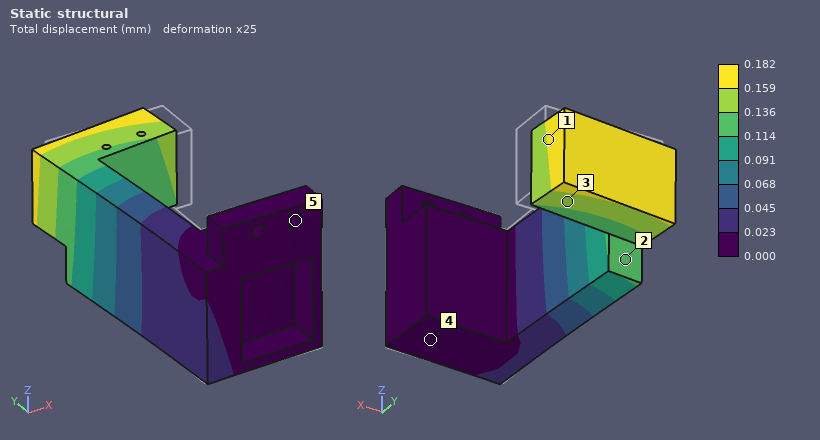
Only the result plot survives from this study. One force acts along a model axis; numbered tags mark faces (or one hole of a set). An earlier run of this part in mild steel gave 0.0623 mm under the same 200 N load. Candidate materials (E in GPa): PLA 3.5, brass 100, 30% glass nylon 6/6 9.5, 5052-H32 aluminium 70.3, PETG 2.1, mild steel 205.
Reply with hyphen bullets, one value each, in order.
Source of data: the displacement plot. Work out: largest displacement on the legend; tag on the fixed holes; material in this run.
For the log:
- 0.182 mm
- 5
- 5052-H32 aluminium
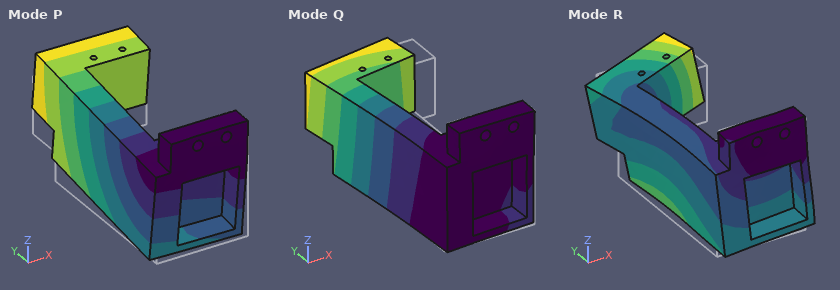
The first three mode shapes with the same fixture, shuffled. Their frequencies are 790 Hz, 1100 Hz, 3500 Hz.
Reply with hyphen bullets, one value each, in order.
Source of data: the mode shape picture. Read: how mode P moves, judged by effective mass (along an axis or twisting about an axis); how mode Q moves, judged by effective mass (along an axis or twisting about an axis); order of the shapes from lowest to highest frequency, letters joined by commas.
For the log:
- along Z
- along X
- P, Q, R
